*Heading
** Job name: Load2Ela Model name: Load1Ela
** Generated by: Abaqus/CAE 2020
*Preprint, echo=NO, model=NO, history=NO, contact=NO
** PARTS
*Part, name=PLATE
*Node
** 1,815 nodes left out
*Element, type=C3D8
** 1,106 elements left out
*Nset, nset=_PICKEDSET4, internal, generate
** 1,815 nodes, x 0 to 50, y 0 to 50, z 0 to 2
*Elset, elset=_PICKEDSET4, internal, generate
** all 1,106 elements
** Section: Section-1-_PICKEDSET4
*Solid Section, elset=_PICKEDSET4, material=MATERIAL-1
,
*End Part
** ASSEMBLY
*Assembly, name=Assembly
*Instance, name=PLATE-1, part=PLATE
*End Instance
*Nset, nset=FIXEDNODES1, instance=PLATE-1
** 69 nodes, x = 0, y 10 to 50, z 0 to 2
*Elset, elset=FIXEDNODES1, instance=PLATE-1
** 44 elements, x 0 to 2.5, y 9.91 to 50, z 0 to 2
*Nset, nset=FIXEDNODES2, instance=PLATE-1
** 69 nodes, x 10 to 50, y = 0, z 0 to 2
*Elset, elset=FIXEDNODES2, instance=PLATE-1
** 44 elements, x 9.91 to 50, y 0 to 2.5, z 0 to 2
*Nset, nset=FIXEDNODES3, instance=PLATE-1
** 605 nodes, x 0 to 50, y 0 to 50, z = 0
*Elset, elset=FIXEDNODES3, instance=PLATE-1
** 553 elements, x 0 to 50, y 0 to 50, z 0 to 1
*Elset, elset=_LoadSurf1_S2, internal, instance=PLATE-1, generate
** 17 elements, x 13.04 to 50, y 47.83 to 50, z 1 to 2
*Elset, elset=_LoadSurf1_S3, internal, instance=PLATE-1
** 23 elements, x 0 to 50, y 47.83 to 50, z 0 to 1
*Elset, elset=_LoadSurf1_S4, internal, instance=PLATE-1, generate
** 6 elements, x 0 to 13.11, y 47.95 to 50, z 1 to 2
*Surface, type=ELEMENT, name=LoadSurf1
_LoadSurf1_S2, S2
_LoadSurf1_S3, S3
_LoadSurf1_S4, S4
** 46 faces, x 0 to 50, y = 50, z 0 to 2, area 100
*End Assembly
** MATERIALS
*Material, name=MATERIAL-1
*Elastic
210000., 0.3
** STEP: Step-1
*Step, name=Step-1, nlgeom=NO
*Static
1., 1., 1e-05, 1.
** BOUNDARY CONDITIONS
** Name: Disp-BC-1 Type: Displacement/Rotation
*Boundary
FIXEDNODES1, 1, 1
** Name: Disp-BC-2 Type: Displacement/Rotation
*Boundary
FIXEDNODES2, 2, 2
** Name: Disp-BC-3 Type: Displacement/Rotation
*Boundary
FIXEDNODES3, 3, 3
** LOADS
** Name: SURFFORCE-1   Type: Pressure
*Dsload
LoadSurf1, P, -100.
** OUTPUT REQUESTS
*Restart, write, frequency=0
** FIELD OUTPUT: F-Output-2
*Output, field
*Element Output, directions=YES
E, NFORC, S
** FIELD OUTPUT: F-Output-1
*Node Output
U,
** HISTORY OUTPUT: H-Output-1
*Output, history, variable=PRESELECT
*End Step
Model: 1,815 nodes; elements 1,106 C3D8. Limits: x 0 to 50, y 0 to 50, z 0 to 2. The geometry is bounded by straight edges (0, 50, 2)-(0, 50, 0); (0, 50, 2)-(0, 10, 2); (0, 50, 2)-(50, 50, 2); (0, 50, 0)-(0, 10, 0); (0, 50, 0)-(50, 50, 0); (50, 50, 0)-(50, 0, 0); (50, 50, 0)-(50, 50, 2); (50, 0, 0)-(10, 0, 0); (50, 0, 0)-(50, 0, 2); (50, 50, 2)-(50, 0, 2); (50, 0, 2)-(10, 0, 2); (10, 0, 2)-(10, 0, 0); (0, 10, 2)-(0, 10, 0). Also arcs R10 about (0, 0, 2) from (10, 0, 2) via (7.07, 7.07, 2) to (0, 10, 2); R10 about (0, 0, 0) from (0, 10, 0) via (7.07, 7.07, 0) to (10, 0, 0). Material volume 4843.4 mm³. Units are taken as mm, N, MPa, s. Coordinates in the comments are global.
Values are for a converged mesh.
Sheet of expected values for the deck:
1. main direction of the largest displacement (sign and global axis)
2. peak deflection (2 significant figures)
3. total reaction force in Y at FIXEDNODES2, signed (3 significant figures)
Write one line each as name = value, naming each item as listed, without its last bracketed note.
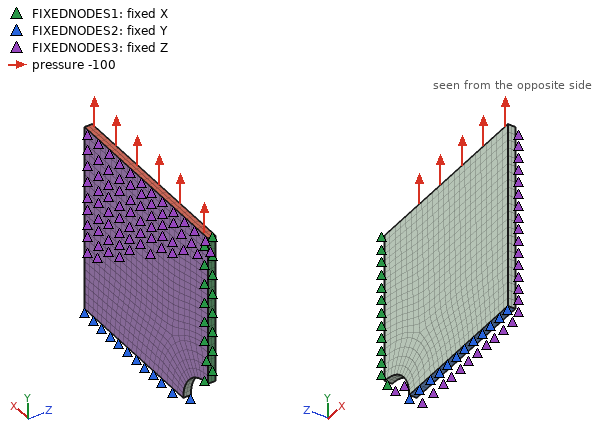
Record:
main direction of the largest displacement = +Y
peak deflection = 0.029 mm
total reaction force in Y at FIXEDNODES2, signed = -10000 N
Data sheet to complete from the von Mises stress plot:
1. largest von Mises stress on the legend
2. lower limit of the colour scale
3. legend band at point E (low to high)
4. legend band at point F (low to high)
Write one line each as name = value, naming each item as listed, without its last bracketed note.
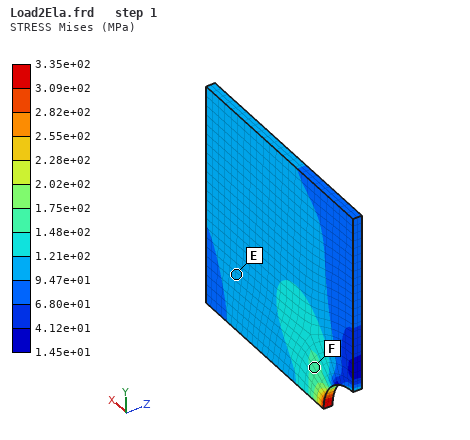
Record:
largest von Mises stress on the legend = 3.35e+02 MPa
lower limit of the colour scale = 1.45e+01 MPa
legend band at point E = 9.47e+01 to 1.21e+02 MPa
legend band at point F = 1.48e+02 to 1.75e+02 MPa
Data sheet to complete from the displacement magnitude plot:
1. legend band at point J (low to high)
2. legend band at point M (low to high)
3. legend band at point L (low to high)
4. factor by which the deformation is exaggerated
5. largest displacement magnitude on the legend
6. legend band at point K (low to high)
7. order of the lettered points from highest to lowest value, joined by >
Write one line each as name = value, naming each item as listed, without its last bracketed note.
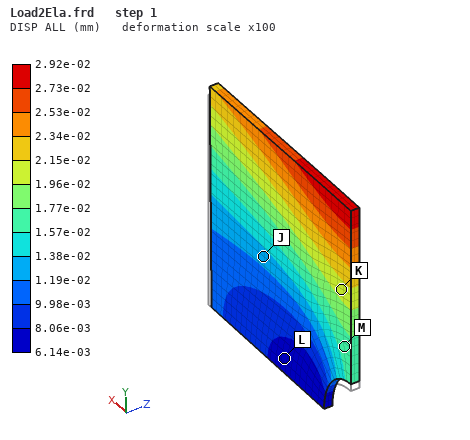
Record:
legend band at point J = 1.19e-02 to 1.38e-02 mm
legend band at point M = 1.57e-02 to 1.77e-02 mm
legend band at point L = 6.14e-03 to 8.06e-03 mm
factor by which the deformation is exaggerated = 100
largest displacement magnitude on the legend = 2.92e-02 mm
legend band at point K = 1.96e-02 to 2.15e-02 mm
order of the lettered points from highest to lowest value, joined by > = K > M > J > L
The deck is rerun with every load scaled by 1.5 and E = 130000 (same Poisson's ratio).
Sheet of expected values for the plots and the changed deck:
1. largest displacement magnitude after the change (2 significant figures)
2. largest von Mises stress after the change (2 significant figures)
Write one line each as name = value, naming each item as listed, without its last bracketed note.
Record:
largest displacement magnitude after the change = 0.071 mm
largest von Mises stress after the change = 500 MPa
